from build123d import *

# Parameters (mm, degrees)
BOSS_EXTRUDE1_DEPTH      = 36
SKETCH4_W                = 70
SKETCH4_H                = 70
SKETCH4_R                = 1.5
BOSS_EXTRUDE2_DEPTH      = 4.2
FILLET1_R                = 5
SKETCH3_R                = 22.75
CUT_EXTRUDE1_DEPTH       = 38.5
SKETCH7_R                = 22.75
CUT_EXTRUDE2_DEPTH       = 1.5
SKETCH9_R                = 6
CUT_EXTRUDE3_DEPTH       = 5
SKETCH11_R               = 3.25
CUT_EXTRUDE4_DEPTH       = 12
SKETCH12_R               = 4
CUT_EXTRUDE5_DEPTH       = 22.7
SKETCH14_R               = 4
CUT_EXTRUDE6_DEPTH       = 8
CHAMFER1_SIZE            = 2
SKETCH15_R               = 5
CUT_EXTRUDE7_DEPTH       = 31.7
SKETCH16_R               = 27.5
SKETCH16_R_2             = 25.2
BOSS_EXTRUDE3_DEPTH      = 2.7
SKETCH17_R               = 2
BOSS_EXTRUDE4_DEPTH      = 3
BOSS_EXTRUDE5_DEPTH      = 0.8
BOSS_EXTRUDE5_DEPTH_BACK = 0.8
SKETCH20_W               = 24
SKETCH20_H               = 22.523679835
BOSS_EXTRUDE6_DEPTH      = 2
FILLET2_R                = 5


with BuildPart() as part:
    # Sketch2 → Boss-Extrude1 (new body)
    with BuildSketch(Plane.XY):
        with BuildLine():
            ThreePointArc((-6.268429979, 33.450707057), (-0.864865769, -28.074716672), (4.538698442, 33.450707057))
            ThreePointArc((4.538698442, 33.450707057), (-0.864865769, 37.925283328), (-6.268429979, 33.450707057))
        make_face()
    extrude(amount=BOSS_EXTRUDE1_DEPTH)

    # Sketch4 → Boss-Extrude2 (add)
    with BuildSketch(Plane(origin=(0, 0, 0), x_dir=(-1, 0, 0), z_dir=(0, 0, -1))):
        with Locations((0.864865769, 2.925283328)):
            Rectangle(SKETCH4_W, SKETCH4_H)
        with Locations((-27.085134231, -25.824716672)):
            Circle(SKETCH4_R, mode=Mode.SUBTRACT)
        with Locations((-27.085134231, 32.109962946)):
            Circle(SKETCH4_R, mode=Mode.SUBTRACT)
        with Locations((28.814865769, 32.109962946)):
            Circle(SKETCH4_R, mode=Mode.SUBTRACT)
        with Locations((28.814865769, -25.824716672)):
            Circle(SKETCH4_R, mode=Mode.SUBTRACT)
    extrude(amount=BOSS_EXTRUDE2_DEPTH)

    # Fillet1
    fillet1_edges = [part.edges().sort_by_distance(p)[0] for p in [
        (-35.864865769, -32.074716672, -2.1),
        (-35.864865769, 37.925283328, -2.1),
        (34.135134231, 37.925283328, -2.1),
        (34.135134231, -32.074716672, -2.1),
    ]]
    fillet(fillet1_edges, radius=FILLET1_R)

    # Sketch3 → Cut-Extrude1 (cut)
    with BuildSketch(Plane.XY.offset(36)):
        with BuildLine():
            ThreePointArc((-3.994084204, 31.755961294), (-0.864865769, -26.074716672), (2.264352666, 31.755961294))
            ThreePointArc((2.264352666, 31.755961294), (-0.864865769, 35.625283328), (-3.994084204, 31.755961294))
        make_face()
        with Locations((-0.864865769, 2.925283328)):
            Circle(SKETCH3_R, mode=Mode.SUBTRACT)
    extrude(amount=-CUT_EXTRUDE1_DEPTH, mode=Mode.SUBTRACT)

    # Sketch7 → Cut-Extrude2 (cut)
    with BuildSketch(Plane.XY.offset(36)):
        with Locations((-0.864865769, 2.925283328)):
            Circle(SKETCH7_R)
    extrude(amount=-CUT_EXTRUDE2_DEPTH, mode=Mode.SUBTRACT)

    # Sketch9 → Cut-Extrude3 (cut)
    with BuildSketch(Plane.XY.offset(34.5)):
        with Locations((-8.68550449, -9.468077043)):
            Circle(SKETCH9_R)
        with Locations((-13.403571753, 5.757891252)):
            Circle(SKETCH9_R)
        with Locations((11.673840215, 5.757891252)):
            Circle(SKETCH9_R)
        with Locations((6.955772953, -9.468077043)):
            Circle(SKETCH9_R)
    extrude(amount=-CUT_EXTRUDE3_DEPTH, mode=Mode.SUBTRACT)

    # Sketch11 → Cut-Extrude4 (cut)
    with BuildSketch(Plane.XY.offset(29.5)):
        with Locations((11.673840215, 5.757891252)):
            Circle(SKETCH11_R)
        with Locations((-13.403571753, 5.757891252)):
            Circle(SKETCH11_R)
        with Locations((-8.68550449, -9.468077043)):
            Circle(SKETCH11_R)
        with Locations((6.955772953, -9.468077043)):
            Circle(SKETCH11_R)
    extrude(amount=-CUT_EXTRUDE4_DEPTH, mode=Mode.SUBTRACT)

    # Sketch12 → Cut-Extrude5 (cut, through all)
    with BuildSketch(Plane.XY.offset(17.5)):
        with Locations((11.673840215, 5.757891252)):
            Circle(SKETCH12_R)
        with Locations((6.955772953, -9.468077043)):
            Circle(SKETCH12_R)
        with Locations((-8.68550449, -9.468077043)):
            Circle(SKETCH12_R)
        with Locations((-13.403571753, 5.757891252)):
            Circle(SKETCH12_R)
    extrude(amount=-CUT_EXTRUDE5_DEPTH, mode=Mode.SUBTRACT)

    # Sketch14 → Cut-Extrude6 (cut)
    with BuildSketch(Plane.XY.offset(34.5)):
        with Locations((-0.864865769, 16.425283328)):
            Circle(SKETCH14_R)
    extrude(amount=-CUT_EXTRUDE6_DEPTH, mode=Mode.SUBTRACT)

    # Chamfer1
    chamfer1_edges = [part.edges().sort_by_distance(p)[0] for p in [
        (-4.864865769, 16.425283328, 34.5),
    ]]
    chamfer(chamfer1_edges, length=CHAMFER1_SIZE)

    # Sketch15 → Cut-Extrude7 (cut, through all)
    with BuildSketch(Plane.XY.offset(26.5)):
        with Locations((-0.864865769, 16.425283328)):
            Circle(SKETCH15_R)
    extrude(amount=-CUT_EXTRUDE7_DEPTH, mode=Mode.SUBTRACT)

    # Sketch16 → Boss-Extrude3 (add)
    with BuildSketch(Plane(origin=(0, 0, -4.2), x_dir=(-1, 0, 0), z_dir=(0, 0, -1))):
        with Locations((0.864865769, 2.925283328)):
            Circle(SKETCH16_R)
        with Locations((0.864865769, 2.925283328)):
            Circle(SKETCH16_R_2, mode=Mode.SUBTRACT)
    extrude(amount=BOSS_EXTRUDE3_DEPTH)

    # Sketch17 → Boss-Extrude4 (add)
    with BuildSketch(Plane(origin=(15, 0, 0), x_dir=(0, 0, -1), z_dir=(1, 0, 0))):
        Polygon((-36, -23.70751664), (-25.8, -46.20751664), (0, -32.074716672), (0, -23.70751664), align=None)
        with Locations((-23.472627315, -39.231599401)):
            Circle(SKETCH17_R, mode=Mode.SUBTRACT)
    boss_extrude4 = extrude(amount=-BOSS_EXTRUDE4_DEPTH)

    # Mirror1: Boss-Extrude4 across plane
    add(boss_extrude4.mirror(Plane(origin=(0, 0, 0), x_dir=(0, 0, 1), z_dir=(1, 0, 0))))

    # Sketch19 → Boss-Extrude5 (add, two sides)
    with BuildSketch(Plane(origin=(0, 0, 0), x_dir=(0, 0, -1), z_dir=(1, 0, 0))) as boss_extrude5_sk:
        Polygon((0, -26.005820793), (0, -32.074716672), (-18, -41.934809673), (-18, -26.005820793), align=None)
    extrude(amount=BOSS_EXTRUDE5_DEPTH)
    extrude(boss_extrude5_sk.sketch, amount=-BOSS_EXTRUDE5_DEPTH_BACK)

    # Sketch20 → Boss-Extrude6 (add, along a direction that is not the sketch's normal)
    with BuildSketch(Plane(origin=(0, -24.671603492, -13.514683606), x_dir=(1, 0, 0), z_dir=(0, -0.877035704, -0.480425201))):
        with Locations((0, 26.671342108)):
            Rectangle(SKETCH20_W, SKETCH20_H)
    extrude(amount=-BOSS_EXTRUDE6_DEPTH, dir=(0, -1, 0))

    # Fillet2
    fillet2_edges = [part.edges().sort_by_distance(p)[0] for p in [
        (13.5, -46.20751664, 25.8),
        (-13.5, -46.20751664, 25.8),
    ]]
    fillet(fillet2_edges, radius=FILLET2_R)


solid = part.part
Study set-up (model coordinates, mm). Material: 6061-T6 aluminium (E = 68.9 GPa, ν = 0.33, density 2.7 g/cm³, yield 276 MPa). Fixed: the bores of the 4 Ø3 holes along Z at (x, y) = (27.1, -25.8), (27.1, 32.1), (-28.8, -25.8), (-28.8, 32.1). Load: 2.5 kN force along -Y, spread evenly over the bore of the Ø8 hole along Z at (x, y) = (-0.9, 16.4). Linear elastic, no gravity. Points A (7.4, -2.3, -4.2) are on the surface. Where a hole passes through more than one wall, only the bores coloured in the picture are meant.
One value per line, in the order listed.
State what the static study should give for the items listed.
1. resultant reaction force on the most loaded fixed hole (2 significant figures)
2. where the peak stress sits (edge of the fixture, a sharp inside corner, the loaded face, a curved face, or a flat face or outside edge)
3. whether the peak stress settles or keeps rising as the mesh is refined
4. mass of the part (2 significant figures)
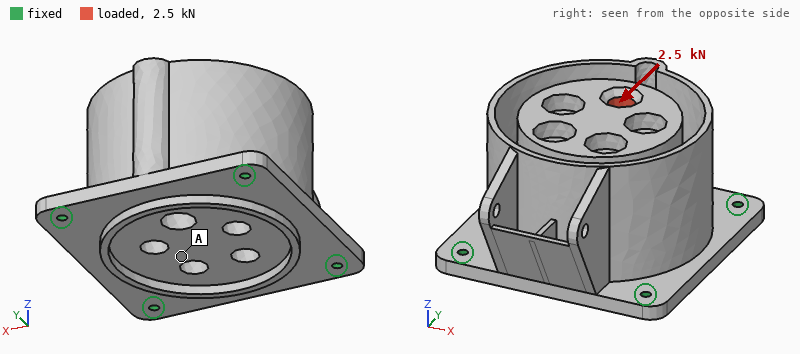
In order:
1.1 kN
edge of the fixture
keeps rising
220 g
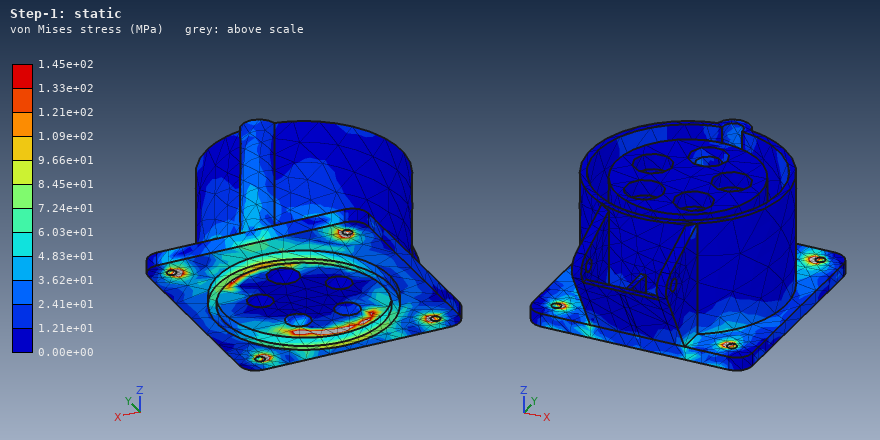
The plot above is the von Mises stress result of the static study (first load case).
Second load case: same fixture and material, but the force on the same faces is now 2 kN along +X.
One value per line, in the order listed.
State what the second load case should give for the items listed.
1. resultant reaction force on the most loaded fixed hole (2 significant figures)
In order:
870 N
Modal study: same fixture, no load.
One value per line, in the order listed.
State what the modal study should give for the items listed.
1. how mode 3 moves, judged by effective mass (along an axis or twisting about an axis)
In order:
along Z
